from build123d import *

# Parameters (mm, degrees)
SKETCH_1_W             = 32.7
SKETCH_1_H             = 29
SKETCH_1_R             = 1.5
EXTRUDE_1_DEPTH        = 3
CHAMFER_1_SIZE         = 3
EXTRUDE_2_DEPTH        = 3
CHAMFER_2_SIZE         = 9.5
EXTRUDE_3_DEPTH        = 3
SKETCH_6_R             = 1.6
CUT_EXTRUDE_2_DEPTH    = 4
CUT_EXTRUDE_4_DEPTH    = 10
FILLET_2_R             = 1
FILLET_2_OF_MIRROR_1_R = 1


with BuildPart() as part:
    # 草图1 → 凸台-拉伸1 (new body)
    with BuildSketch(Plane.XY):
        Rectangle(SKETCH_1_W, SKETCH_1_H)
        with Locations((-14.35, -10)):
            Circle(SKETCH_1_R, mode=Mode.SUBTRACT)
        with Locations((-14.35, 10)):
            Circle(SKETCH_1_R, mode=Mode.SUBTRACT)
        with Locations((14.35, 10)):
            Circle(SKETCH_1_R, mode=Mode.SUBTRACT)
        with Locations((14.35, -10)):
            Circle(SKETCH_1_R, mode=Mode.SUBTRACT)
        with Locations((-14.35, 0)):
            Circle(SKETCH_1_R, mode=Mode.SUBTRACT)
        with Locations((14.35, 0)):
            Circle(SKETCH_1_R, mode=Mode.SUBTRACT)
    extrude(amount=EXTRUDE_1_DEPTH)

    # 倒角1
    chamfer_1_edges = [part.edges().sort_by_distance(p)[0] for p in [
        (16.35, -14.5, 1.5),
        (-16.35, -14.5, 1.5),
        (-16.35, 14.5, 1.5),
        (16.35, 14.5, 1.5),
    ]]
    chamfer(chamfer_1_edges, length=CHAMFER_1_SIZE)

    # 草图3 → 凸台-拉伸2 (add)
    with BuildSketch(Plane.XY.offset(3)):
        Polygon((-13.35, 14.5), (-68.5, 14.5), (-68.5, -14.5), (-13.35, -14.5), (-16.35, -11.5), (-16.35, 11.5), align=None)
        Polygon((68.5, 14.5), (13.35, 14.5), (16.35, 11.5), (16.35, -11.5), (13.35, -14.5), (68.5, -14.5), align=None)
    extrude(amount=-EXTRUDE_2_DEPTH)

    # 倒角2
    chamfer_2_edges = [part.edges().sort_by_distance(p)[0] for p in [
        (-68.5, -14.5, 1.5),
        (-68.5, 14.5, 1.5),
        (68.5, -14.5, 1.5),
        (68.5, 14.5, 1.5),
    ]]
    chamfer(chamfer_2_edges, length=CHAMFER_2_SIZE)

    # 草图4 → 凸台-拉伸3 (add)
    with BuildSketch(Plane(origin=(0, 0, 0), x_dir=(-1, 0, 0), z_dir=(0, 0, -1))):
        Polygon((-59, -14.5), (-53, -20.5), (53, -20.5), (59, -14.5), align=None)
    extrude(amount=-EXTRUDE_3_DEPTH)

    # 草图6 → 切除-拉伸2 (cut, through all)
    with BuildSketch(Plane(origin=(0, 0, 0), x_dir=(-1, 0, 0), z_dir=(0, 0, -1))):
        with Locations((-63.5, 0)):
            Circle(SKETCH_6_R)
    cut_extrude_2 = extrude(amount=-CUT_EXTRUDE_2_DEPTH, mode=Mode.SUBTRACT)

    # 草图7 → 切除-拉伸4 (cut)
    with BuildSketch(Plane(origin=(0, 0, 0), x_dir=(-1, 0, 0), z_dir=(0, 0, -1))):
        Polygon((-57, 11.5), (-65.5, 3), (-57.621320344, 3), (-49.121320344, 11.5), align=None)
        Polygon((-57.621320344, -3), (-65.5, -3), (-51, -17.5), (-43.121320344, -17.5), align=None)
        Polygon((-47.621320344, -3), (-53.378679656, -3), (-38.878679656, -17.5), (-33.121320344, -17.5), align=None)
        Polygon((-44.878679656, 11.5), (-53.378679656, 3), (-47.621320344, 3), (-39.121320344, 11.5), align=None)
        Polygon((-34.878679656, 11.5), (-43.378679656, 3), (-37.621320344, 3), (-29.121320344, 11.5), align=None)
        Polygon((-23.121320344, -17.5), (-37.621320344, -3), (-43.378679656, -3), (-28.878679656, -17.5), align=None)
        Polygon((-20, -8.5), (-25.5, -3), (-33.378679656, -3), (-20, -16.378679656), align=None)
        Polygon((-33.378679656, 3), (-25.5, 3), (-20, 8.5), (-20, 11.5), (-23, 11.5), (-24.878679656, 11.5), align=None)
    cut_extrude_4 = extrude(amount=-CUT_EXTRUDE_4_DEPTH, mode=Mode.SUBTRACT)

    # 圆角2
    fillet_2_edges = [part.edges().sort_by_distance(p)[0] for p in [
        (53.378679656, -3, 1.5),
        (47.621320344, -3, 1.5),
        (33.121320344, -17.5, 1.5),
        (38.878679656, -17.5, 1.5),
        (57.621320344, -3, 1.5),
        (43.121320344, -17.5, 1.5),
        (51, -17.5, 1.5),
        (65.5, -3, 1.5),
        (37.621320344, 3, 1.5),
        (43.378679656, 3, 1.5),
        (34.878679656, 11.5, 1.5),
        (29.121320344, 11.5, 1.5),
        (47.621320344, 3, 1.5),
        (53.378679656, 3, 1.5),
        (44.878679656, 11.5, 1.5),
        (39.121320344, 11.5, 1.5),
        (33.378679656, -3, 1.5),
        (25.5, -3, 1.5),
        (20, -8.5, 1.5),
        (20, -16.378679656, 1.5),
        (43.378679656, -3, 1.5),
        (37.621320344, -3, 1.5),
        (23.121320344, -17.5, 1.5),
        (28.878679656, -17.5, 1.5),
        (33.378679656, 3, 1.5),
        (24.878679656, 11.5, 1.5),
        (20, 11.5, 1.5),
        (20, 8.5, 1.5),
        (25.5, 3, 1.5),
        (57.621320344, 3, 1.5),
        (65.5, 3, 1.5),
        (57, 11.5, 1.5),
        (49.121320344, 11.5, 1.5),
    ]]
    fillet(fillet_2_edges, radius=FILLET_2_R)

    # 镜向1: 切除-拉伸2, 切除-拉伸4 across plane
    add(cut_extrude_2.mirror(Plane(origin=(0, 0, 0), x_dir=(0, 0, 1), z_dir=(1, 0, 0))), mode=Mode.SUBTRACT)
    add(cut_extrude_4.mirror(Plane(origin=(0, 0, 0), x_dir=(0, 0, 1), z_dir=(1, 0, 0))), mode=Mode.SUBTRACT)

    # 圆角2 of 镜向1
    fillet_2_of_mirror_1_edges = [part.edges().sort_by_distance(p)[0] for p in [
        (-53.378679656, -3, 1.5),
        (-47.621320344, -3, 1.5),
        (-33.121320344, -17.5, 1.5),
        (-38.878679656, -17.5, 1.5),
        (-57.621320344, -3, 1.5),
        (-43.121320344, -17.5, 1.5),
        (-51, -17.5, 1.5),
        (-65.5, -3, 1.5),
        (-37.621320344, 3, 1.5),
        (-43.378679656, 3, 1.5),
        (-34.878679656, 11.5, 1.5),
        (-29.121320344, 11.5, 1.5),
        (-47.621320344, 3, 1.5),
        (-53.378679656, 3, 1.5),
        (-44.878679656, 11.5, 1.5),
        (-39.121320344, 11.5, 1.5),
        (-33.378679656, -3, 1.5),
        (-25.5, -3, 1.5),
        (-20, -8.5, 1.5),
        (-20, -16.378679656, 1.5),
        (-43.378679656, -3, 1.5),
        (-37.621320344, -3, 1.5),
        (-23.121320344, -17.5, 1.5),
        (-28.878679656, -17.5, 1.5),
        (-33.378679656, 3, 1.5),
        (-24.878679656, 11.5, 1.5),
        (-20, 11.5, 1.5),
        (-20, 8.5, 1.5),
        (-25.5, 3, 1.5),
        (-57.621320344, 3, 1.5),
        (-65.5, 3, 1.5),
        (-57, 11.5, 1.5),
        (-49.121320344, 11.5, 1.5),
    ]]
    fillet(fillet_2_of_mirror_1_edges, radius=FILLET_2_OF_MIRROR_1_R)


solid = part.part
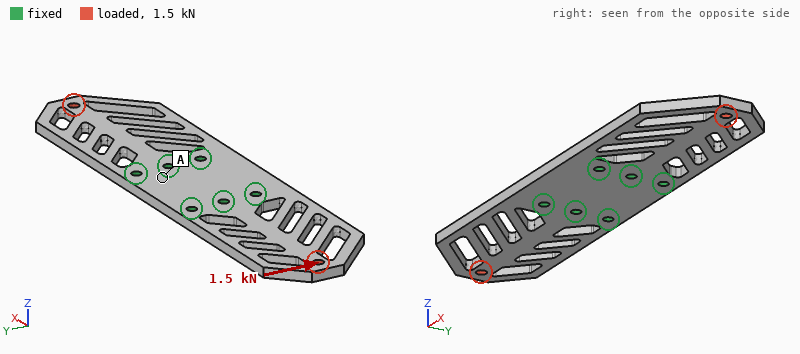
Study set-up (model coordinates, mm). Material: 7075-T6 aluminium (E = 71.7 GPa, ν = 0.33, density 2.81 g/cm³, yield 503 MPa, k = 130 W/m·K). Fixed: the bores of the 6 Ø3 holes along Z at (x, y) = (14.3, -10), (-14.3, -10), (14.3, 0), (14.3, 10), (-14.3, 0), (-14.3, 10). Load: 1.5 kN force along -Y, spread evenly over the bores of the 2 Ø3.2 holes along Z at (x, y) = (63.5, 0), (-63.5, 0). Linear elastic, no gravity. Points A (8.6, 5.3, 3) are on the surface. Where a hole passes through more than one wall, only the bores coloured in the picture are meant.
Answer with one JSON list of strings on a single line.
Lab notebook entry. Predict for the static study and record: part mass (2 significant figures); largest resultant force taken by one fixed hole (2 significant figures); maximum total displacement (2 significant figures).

["28 g", "1.2 kN", "0.23 mm"]
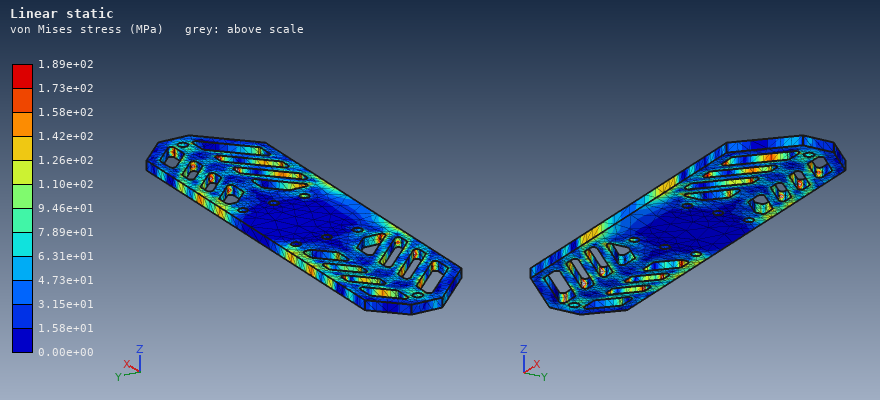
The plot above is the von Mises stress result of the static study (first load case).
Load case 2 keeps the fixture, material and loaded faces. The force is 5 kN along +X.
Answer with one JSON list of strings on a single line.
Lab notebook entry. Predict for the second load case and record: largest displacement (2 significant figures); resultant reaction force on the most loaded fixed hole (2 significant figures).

["70 µm", "980 N"]
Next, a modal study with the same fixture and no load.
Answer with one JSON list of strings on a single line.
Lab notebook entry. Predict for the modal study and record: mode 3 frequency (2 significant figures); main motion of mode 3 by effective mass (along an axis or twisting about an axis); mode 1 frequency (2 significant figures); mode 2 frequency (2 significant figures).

["2800 Hz", "twisting about X", "900 Hz", "910 Hz"]
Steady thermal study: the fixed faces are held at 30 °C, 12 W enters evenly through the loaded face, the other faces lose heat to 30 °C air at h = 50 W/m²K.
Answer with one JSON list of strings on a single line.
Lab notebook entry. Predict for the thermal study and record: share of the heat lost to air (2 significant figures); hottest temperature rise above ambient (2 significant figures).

["45 %", "38 K"]
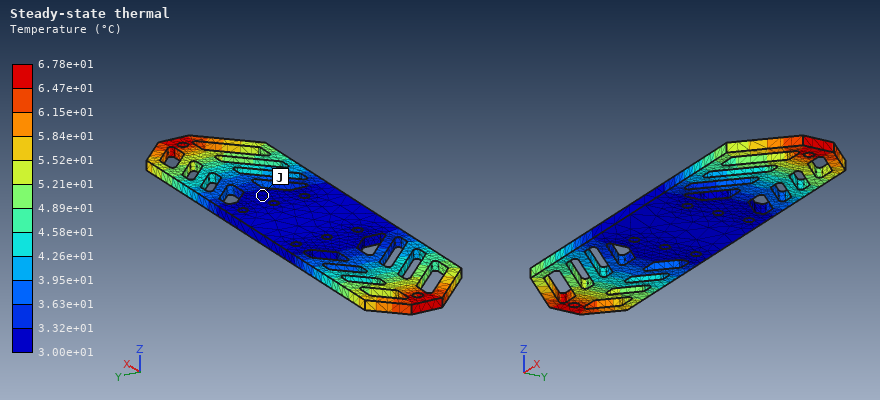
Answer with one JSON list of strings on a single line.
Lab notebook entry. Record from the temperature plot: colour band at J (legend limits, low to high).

["3.00e+01 to 3.32e+01 °C"]
